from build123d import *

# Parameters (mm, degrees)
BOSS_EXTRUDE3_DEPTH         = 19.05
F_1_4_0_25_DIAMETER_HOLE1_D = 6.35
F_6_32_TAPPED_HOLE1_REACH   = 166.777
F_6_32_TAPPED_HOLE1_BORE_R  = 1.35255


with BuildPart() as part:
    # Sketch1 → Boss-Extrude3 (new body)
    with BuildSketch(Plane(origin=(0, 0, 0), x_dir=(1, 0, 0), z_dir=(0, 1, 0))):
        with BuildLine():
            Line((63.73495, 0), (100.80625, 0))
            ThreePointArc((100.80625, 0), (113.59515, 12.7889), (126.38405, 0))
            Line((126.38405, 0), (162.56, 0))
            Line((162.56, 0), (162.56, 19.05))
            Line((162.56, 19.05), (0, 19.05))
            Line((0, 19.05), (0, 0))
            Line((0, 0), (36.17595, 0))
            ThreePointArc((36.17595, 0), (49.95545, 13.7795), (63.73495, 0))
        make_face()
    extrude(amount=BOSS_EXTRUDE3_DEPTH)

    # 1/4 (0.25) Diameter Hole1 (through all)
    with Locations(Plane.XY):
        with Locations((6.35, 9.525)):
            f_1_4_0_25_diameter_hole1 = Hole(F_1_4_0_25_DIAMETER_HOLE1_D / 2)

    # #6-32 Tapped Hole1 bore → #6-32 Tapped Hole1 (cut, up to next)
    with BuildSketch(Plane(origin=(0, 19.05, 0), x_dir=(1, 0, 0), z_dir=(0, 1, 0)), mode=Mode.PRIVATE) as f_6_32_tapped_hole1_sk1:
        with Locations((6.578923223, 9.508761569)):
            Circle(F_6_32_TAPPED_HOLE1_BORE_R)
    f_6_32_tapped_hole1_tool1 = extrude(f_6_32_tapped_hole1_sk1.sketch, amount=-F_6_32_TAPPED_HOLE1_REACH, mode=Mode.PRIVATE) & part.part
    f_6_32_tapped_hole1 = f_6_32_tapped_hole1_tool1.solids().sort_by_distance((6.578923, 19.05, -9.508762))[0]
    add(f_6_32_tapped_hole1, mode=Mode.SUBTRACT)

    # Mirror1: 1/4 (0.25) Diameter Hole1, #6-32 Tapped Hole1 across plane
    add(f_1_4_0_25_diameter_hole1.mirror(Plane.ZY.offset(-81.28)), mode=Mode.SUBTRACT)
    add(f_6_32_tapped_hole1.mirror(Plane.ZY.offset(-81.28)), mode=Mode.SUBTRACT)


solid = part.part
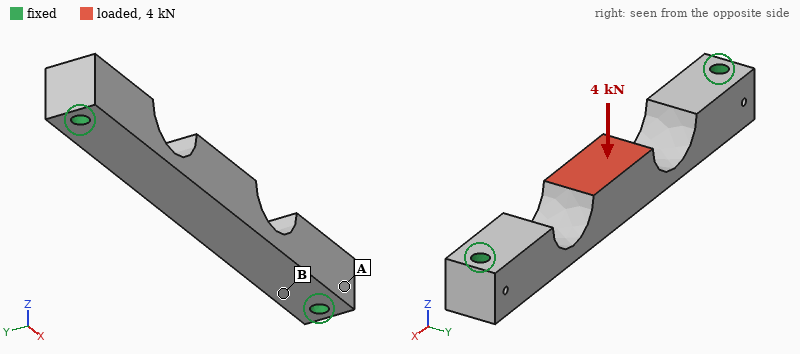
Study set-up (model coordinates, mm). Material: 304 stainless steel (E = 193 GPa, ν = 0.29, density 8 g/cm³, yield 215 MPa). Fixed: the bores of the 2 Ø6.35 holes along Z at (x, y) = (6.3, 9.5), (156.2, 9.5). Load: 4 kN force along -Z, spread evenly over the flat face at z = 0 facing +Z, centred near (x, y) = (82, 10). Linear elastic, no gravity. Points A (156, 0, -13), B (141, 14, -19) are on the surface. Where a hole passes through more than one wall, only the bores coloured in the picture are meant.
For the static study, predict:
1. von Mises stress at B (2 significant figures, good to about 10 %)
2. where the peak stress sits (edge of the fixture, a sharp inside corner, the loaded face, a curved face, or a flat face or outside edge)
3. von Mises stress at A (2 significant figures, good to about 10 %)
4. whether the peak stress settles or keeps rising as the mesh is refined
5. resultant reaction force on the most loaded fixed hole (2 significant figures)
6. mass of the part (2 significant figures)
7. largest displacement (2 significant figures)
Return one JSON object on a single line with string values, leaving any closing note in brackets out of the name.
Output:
{"von Mises stress at B": "41 MPa", "where the peak stress sits": "edge of the fixture", "von Mises stress at A": "16 MPa", "whether the peak stress settles or keeps rising as the mesh is refined": "keeps rising", "resultant reaction force on the most loaded fixed hole": "2.3 kN", "mass of the part": "380 g", "largest displacement": "58 µm"}
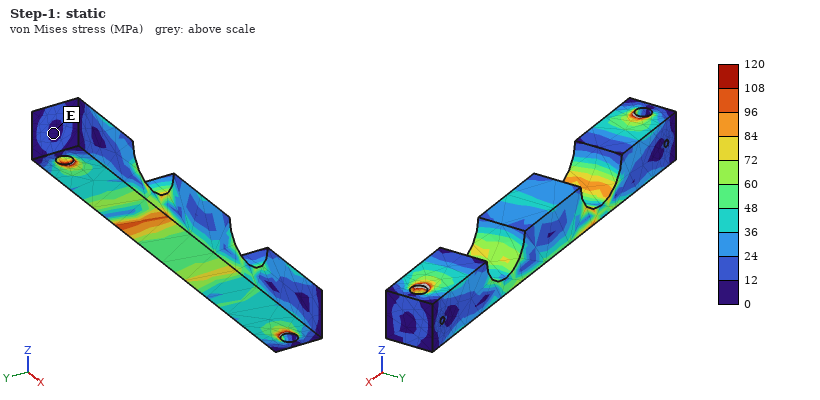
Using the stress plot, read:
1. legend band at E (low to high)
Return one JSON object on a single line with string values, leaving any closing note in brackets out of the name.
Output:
{"legend band at E": "0 to 12 MPa"}
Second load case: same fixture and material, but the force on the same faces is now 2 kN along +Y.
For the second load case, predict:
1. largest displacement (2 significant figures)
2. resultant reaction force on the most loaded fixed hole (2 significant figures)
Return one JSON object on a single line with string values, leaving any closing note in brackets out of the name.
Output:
{"largest displacement": "77 µm", "resultant reaction force on the most loaded fixed hole": "1.0 kN"}
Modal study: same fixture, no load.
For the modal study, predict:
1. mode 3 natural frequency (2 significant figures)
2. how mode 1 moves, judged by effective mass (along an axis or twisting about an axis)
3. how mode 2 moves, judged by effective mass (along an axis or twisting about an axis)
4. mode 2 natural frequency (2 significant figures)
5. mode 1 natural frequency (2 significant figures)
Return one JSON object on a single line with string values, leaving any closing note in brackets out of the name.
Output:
{"mode 3 natural frequency": "6100 Hz", "how mode 1 moves, judged by effective mass": "along Y", "how mode 2 moves, judged by effective mass": "along Z", "mode 2 natural frequency": "3600 Hz", "mode 1 natural frequency": "3100 Hz"}
